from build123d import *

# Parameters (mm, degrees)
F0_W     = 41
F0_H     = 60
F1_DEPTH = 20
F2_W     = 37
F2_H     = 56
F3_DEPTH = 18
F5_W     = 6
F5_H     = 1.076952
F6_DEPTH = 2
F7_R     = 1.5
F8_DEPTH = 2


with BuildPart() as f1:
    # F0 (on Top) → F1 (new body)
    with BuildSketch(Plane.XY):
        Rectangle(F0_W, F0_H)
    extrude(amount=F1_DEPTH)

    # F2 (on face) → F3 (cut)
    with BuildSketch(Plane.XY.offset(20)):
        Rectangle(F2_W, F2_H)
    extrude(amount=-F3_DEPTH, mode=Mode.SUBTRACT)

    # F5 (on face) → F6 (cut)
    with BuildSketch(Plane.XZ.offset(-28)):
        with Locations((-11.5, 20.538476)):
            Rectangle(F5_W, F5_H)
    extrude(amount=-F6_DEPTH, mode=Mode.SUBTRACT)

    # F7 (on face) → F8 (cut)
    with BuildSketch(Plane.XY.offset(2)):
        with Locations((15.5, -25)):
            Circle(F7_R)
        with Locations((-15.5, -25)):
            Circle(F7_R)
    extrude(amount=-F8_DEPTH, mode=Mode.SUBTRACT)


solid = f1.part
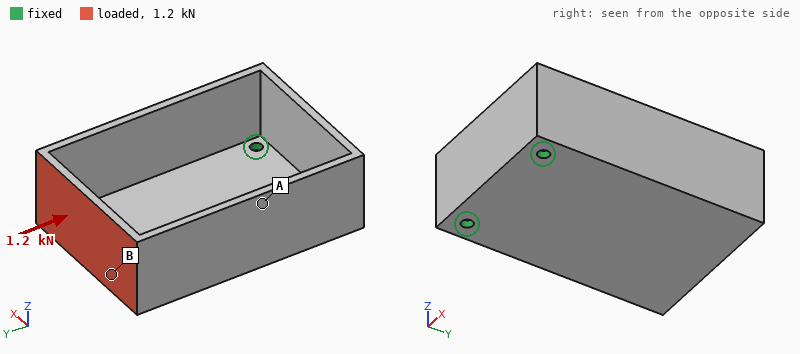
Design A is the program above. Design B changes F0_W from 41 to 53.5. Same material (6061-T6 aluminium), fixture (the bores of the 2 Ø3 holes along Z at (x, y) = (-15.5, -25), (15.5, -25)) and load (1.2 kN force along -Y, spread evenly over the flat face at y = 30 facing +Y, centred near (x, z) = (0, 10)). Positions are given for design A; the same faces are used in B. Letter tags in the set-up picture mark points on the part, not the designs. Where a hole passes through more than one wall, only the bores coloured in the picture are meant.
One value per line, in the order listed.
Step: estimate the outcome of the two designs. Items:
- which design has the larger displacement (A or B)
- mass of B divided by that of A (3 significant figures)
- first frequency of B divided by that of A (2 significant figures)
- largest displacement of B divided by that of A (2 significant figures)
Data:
A
2.26
0.72
0.82
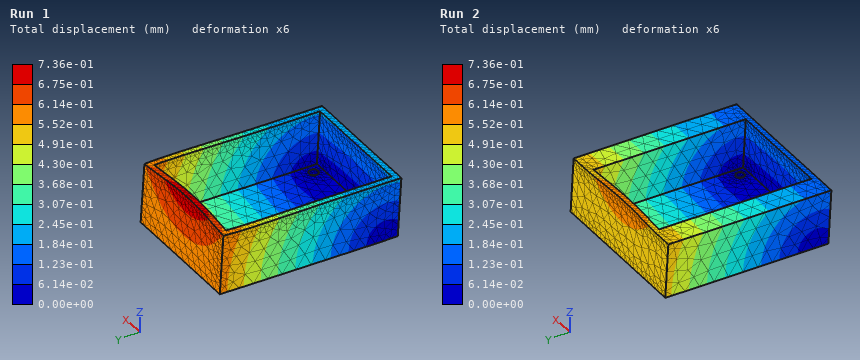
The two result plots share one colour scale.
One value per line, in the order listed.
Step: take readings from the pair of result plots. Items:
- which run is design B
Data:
Run 2
